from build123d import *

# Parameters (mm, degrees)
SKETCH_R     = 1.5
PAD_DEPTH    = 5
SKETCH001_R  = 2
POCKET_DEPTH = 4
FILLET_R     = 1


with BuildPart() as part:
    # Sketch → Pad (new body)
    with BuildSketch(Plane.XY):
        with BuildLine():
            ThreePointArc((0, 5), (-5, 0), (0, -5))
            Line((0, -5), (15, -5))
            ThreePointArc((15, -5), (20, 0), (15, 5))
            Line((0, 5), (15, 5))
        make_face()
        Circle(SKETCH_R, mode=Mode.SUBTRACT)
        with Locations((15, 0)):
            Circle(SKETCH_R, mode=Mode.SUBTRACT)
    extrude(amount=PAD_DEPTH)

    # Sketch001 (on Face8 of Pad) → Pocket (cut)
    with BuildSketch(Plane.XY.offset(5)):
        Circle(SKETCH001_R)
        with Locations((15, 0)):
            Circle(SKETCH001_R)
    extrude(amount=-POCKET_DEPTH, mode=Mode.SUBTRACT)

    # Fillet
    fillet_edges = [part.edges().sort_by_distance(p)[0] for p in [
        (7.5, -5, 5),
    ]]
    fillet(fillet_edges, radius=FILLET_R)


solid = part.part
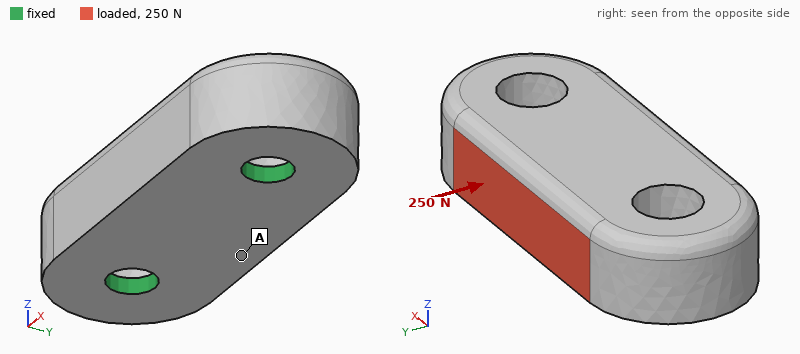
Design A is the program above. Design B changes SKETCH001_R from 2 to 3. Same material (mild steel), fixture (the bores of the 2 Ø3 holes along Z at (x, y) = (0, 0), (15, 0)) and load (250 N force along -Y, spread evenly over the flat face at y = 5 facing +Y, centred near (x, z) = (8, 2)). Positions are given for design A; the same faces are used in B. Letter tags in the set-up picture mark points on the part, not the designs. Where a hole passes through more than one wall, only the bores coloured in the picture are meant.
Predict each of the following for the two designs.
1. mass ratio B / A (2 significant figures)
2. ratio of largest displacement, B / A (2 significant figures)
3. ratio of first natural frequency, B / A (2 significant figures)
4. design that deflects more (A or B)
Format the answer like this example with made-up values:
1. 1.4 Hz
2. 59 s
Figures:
1. 0.88
2. 1.6
3. 0.83
4. B
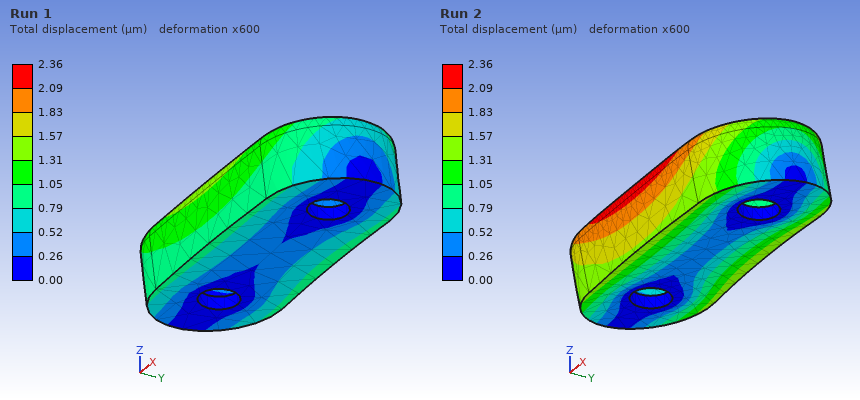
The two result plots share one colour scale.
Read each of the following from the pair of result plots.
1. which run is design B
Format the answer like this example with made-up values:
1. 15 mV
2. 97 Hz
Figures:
1. Run 2
